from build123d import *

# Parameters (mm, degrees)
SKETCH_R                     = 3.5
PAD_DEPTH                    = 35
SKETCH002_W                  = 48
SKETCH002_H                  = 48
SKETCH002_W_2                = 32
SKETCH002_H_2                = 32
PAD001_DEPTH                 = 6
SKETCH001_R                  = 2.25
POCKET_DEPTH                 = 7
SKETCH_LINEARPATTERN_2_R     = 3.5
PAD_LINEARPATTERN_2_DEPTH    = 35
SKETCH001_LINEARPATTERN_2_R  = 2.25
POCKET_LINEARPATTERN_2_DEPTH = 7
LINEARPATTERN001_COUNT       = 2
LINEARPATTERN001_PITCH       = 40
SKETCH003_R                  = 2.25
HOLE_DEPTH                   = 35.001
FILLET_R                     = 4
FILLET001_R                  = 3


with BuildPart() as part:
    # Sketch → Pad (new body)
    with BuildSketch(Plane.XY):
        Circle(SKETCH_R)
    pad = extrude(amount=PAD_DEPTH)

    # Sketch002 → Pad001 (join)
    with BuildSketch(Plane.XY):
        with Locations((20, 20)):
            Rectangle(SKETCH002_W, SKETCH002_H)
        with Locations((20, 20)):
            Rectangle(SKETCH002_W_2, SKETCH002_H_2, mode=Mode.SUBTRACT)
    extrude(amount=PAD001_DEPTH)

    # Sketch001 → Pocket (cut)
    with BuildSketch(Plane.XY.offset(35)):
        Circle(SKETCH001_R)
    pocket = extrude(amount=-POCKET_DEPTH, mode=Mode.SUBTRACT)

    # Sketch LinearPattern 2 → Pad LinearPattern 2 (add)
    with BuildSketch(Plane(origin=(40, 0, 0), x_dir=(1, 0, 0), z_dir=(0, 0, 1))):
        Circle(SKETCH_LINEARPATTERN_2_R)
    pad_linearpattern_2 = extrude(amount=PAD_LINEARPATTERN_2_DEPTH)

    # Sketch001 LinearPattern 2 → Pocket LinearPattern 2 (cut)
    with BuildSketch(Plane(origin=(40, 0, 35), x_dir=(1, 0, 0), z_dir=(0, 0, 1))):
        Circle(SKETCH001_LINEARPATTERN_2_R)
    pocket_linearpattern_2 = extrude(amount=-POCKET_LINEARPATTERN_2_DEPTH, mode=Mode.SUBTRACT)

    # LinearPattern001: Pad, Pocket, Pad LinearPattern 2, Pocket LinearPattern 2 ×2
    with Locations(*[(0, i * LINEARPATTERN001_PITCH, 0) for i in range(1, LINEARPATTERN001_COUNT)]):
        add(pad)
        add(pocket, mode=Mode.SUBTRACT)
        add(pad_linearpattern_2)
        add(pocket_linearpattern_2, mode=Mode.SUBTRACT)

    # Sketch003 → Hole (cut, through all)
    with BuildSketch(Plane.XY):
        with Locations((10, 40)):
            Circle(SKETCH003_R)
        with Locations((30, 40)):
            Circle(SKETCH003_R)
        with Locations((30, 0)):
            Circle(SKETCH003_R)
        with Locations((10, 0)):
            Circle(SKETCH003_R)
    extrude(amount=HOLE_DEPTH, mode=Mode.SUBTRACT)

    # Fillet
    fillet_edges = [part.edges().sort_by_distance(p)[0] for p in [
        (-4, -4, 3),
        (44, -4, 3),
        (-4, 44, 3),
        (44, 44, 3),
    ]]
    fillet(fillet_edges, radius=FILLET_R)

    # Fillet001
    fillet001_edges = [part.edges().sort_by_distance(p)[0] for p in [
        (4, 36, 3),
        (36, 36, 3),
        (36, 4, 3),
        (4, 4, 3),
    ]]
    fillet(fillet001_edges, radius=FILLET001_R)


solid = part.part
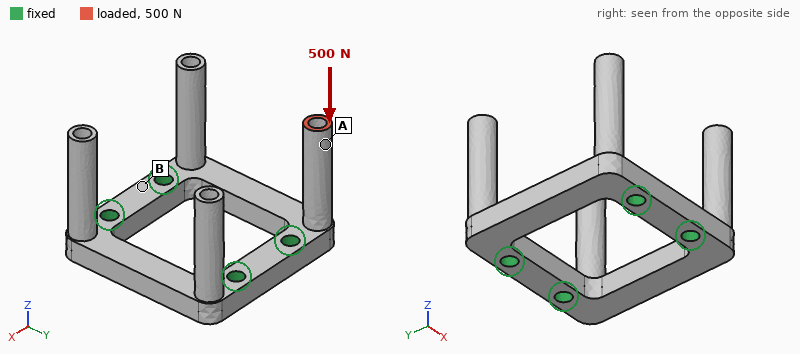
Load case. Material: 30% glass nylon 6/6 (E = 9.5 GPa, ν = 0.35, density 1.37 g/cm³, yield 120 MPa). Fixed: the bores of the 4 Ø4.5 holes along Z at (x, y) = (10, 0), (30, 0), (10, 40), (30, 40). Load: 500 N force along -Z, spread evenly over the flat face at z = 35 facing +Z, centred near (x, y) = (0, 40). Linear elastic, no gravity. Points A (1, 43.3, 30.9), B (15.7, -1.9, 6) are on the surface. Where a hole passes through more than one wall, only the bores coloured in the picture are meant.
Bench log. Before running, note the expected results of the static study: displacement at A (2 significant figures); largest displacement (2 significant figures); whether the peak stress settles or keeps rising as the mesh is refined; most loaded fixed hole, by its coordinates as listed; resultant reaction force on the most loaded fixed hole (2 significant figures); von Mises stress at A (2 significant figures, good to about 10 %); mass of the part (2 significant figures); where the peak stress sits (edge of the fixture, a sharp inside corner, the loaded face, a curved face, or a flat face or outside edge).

0.36 mm
0.43 mm
keeps rising
(10, 40)
500 N
22 MPa
15 g
edge of the fixture
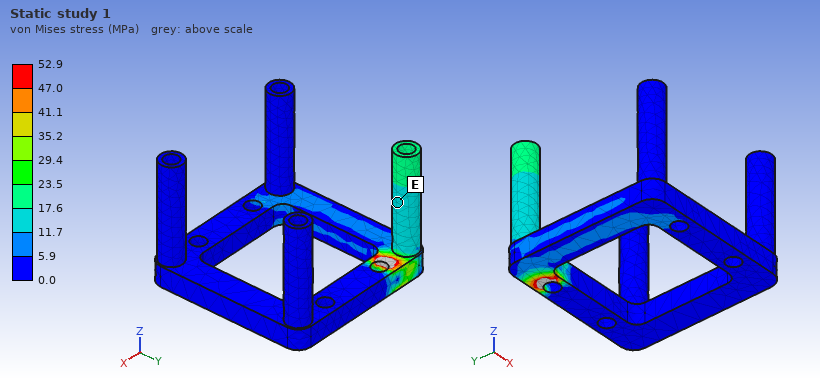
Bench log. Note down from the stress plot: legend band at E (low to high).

11.7 to 17.6 MPa
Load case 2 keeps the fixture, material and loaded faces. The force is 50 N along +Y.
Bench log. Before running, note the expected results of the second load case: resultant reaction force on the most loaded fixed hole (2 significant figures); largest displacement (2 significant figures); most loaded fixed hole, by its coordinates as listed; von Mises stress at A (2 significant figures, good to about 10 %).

39 N
0.61 mm
(10, 40)
7.2 MPa
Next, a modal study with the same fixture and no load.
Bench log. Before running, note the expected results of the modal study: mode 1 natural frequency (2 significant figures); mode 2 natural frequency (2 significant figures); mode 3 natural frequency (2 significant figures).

2300 Hz
2300 Hz
2400 Hz
